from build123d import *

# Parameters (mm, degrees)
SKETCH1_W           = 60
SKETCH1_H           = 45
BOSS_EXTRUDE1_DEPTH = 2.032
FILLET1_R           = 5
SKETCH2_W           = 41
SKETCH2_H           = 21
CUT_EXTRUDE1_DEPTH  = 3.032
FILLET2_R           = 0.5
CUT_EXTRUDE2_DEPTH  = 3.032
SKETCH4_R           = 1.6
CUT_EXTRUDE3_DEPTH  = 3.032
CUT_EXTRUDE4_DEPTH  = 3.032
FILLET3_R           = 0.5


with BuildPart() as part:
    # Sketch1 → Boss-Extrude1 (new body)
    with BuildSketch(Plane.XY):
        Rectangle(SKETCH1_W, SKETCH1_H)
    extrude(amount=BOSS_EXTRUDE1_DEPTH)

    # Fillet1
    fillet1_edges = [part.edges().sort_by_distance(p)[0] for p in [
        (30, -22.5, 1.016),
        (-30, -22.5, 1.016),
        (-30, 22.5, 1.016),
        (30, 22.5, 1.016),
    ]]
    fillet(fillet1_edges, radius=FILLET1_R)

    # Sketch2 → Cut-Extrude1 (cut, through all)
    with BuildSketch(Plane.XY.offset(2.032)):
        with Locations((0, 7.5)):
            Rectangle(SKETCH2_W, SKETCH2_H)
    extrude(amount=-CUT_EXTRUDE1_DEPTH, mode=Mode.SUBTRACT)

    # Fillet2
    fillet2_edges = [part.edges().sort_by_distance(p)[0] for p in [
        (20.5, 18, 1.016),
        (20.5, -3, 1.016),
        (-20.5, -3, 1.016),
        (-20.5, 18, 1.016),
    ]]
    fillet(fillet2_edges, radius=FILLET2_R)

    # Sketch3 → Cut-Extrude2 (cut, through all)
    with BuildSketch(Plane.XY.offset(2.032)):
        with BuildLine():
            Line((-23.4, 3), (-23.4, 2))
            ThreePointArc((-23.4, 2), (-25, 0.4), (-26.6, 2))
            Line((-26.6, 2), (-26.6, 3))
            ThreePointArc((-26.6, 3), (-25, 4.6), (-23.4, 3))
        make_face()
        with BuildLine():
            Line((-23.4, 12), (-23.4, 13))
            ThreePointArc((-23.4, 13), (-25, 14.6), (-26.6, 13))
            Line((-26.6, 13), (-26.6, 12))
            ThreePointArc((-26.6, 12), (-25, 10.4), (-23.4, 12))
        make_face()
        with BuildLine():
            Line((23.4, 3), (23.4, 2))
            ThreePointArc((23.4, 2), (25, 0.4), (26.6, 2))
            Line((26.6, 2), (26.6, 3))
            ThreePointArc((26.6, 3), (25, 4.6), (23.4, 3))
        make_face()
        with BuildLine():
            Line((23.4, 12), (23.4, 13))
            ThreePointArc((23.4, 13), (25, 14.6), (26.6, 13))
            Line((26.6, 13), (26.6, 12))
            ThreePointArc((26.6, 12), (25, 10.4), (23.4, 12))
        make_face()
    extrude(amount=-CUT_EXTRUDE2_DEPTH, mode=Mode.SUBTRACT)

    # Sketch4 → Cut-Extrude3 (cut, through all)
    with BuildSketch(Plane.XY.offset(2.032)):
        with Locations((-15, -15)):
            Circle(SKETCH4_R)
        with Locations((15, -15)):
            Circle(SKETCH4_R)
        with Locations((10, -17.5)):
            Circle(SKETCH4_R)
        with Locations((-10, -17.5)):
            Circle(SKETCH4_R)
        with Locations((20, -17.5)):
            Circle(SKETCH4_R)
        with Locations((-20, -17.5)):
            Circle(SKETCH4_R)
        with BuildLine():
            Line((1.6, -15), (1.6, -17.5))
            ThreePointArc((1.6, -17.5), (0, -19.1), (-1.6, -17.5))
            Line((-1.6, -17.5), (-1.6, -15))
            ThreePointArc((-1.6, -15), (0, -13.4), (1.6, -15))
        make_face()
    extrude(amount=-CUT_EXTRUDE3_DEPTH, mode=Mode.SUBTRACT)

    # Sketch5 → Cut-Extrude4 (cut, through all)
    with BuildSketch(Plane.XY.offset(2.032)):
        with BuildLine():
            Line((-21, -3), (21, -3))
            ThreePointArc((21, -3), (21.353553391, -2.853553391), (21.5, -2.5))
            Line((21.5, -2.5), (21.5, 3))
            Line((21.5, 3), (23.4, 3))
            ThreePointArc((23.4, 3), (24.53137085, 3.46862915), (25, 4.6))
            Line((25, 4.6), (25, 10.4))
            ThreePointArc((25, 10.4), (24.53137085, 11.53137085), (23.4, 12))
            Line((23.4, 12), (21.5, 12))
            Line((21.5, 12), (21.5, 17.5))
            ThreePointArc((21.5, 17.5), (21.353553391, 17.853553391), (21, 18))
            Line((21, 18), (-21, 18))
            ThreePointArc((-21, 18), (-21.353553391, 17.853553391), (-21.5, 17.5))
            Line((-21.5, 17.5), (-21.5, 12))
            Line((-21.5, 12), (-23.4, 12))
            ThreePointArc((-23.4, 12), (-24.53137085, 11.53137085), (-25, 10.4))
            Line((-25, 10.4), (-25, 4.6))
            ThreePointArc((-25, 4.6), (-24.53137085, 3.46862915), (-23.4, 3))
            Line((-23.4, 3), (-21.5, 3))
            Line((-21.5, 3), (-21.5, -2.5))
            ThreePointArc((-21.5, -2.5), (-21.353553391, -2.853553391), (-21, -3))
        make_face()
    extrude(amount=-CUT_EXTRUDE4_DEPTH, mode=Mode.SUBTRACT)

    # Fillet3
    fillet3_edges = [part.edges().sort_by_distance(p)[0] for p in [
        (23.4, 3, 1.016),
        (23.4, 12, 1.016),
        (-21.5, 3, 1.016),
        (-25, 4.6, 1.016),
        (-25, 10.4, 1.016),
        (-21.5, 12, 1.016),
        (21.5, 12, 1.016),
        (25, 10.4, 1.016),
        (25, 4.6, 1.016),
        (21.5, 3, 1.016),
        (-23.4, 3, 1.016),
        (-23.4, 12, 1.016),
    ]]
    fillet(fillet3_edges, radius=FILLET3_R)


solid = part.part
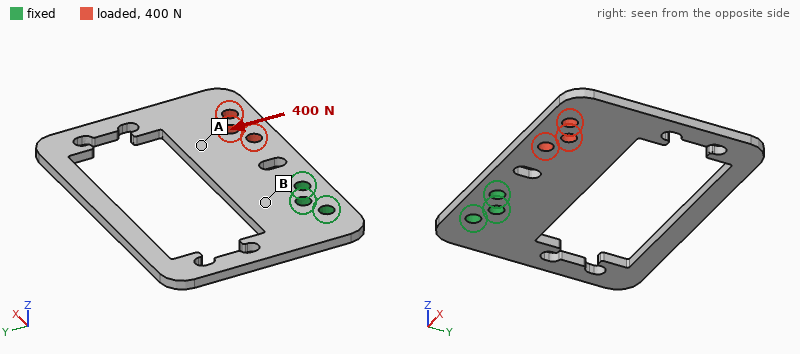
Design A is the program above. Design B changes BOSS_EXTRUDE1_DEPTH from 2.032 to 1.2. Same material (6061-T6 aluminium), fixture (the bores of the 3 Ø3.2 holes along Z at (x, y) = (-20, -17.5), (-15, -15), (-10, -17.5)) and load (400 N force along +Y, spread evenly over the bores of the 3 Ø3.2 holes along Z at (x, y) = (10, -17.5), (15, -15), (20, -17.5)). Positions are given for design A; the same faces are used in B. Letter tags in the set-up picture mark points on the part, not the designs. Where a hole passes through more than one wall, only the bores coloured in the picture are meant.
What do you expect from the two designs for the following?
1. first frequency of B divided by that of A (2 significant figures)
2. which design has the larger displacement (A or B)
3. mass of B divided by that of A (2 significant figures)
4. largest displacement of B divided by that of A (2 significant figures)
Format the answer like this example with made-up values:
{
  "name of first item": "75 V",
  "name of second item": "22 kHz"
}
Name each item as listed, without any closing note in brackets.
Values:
{
  "first frequency of B divided by that of A": "0.60",
  "which design has the larger displacement": "B",
  "mass of B divided by that of A": "0.59",
  "largest displacement of B divided by that of A": "1.7"
}
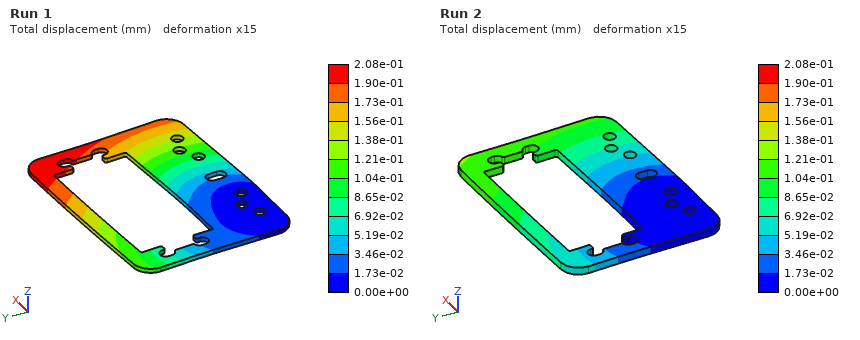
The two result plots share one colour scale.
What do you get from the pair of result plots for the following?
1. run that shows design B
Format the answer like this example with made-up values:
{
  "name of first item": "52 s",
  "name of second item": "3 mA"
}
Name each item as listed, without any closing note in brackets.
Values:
{
  "run that shows design B": "Run 1"
}
